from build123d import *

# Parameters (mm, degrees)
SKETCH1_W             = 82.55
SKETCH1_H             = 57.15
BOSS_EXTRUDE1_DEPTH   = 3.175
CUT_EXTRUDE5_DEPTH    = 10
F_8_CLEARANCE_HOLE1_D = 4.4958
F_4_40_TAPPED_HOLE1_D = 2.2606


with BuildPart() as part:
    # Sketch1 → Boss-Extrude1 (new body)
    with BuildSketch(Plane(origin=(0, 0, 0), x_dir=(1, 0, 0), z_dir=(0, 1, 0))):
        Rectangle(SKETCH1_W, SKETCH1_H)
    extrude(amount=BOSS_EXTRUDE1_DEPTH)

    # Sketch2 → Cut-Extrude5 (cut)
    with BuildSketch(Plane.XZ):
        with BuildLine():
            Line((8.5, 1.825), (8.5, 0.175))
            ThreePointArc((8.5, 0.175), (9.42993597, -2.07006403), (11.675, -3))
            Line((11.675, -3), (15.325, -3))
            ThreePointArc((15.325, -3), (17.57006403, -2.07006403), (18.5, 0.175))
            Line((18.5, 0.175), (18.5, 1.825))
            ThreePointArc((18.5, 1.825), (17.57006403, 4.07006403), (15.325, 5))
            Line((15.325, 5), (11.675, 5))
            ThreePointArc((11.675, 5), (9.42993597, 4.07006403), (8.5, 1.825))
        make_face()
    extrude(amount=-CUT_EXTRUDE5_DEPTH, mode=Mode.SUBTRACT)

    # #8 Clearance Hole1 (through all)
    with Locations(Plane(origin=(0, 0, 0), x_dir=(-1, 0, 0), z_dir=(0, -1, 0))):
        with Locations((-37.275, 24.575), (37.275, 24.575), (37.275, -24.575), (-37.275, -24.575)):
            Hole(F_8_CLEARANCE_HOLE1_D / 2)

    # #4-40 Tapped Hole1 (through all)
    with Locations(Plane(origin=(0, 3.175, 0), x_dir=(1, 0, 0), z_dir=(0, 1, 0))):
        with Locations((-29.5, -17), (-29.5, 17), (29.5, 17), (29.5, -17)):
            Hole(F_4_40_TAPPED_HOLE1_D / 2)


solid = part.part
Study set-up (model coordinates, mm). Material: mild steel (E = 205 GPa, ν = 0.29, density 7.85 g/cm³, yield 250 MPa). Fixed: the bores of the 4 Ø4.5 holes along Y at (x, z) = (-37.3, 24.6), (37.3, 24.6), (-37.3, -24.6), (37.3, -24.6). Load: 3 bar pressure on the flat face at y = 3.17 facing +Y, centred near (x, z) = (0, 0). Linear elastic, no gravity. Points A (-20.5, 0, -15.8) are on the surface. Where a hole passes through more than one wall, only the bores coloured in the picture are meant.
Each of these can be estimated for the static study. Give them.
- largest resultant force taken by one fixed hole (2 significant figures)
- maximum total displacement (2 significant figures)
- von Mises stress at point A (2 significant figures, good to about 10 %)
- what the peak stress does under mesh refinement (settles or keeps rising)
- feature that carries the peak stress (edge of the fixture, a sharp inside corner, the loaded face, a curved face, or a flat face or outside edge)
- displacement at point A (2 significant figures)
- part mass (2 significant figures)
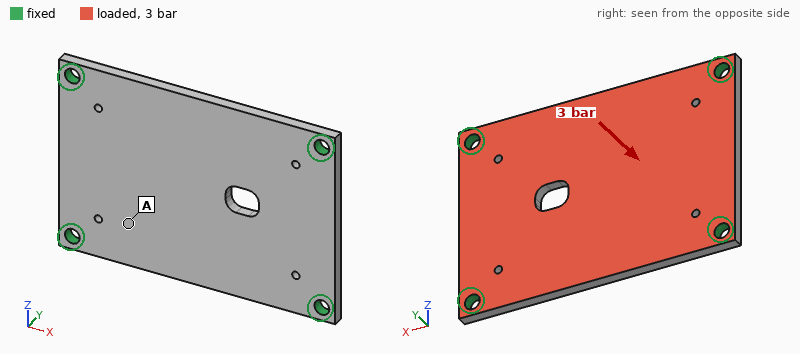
340 N
66 µm
17 MPa
keeps rising
edge of the fixture
35 µm
110 g
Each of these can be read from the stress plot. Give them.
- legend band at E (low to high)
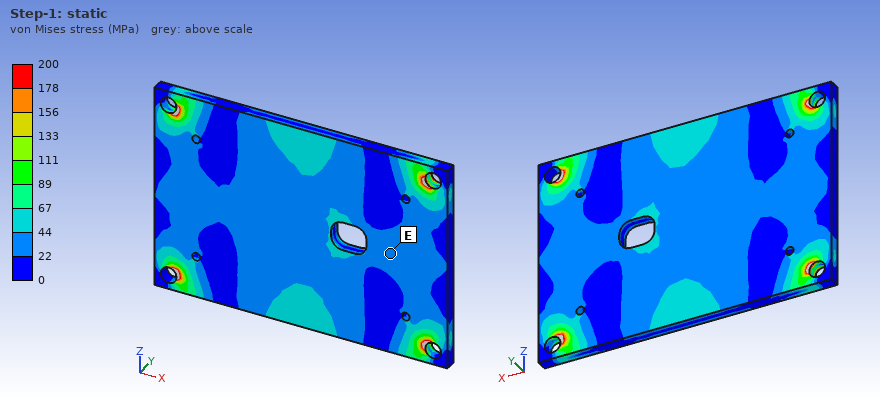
22 to 44 MPa
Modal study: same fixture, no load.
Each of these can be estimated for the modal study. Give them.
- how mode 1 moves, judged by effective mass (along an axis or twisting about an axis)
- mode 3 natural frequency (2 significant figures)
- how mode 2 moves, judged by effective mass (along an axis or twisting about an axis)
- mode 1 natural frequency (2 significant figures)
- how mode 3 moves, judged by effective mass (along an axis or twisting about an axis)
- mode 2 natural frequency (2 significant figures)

along Y
6100 Hz
twisting about X
2500 Hz
twisting about Z
4000 Hz
